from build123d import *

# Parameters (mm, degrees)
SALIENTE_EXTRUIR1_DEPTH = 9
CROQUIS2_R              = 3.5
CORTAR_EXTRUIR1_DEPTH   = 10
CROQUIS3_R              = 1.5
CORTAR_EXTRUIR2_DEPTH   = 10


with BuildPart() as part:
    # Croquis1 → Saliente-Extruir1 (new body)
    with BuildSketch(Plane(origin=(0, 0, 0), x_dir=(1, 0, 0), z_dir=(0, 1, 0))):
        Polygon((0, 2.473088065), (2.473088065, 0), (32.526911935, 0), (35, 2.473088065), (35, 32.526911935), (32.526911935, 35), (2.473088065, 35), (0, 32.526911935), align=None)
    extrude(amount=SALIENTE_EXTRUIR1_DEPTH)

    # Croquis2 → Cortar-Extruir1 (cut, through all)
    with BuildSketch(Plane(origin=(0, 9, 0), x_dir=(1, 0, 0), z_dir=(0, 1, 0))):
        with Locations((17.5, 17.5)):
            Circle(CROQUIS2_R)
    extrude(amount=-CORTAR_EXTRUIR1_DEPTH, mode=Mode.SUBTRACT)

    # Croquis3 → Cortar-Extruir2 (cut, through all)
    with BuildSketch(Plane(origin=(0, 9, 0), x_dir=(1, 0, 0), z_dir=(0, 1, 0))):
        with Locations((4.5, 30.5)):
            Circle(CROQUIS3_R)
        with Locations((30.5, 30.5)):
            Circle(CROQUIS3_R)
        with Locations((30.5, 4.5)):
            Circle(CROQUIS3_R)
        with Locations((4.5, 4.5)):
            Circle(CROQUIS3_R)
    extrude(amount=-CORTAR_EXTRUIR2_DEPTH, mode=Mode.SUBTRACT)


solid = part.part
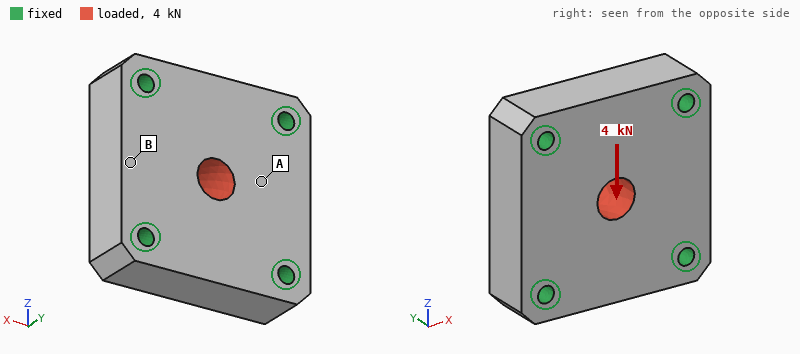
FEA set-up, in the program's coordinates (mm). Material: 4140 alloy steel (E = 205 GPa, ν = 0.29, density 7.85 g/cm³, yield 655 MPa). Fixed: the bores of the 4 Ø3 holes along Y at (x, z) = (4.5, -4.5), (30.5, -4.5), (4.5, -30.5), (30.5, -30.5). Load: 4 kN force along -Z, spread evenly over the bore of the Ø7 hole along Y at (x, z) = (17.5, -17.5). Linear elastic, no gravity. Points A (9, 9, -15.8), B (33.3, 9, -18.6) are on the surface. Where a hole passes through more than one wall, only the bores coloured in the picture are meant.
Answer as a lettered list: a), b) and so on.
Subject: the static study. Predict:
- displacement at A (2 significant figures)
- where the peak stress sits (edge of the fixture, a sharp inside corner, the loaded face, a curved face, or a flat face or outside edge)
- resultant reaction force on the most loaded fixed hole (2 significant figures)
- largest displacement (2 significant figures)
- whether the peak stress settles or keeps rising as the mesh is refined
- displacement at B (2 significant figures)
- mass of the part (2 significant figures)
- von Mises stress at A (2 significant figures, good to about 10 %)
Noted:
a) 0.62 µm
b) edge of the fixture
c) 1.1 kN
d) 1.5 µm
e) keeps rising
f) 0.23 µm
g) 81 g
h) 10 MPa
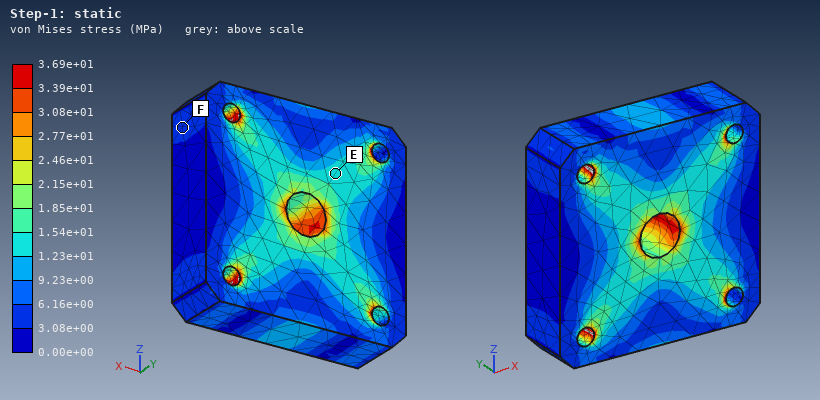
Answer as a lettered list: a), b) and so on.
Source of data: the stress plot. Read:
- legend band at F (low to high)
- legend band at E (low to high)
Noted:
a) 3.08e+00 to 6.16e+00 MPa
b) 1.23e+01 to 1.54e+01 MPa
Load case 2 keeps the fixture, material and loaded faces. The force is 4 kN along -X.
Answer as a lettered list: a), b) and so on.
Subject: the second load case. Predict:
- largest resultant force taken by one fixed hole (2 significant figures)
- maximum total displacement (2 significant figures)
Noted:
a) 1.1 kN
b) 1.5 µm
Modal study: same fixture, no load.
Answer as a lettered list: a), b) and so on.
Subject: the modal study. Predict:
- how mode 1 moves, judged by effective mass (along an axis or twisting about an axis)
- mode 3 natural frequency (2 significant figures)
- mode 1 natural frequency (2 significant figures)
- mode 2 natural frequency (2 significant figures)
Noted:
a) along Y
b) 46 kHz
c) 33 kHz
d) 46 kHz
